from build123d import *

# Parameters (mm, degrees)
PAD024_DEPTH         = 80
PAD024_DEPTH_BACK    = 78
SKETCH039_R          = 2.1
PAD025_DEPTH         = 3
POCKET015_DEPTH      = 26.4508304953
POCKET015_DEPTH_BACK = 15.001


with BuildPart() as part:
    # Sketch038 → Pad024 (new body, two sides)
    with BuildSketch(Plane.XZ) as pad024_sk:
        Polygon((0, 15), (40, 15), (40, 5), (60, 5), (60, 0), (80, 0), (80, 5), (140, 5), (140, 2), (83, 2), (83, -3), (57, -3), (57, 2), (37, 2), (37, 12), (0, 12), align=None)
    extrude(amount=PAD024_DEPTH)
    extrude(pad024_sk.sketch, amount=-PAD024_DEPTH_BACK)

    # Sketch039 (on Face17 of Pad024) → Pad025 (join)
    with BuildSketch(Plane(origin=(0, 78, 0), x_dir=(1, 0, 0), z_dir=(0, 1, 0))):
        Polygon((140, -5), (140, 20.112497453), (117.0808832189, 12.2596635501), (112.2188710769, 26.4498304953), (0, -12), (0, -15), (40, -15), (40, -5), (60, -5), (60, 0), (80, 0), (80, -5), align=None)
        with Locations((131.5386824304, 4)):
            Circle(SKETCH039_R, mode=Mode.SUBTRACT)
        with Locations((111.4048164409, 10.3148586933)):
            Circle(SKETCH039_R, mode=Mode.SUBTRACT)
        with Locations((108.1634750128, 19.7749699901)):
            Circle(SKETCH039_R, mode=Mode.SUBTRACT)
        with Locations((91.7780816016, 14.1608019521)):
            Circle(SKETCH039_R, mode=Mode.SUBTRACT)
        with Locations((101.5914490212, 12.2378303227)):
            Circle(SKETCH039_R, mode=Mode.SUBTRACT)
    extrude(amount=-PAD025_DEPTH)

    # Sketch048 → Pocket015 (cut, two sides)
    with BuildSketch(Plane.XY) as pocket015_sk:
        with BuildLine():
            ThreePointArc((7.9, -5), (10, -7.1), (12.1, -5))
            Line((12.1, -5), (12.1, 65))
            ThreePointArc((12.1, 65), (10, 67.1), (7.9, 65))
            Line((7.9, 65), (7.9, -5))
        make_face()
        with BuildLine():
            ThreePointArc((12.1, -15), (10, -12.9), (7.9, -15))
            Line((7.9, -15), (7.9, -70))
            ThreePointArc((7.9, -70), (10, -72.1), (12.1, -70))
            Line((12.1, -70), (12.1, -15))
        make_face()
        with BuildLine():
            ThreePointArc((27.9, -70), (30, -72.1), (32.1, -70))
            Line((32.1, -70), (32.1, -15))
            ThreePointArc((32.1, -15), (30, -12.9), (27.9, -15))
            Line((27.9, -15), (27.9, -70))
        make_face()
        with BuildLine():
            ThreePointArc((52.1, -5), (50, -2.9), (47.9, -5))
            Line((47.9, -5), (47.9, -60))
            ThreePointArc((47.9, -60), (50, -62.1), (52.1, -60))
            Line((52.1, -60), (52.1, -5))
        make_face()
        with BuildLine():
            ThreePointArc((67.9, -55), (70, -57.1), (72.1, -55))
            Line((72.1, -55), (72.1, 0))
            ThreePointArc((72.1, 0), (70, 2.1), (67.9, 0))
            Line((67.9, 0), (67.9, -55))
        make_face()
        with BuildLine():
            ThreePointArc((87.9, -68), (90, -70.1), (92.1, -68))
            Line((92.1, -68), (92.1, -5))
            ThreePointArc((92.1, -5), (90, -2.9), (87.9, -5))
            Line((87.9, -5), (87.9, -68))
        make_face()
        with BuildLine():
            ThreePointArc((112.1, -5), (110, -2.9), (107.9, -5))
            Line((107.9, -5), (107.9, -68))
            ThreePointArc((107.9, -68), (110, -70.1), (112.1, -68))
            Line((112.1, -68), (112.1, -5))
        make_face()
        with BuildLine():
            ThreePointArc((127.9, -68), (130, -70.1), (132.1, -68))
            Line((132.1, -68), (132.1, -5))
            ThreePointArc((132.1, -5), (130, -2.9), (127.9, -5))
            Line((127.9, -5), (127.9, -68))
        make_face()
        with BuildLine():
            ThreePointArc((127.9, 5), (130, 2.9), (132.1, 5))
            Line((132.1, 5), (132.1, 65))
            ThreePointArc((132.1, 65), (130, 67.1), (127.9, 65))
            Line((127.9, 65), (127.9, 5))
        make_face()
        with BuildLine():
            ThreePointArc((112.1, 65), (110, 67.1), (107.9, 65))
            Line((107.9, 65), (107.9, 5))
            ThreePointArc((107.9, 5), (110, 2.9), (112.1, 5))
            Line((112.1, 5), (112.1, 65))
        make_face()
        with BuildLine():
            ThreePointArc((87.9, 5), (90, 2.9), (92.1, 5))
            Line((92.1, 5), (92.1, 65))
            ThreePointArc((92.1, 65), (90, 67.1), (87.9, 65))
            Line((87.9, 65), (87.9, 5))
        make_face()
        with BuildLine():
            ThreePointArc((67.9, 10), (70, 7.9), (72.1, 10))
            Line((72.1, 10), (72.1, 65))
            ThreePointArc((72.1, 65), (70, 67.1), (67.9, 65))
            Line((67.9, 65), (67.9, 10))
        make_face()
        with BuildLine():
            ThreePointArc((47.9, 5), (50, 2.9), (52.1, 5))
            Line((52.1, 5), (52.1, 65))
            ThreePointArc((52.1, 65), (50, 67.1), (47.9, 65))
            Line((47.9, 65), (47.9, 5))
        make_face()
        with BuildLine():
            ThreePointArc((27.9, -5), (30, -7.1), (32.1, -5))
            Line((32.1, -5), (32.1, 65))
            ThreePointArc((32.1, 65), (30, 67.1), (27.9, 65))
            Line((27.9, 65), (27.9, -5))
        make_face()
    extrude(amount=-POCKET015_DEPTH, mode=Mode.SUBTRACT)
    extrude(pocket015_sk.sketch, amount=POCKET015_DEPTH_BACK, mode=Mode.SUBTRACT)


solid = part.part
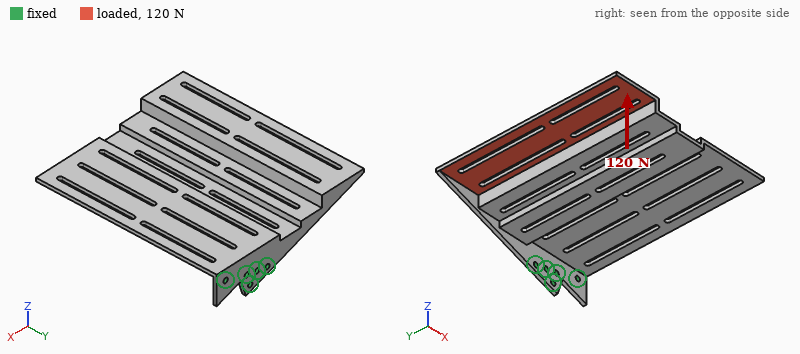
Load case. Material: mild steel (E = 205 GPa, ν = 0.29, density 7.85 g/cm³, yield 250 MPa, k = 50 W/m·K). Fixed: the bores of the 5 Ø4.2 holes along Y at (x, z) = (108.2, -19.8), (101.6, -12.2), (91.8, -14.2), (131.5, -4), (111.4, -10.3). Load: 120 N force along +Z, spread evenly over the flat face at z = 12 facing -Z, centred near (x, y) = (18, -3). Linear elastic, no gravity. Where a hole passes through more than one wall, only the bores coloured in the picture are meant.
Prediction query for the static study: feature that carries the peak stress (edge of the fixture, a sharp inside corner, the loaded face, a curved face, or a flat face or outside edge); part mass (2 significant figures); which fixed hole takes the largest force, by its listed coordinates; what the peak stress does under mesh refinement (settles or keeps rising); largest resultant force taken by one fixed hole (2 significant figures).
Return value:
edge of the fixture
550 g
(91.8, -14.2)
keeps rising
530 N
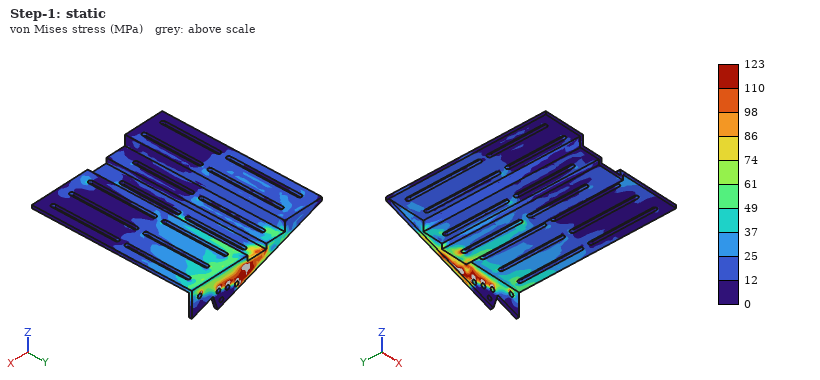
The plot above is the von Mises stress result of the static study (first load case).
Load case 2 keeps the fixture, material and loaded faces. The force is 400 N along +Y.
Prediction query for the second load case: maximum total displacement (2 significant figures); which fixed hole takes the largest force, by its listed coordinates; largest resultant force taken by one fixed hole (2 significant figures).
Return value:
1.7 mm
(131.5, -4)
860 N
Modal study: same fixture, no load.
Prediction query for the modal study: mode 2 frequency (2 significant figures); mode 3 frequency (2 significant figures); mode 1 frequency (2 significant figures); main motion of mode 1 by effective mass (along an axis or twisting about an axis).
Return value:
240 Hz
320 Hz
82 Hz
along Z
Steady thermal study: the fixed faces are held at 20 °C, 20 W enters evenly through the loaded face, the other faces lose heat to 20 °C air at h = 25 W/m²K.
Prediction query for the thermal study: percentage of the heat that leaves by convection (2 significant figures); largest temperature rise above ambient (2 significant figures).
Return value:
95 %
69 K
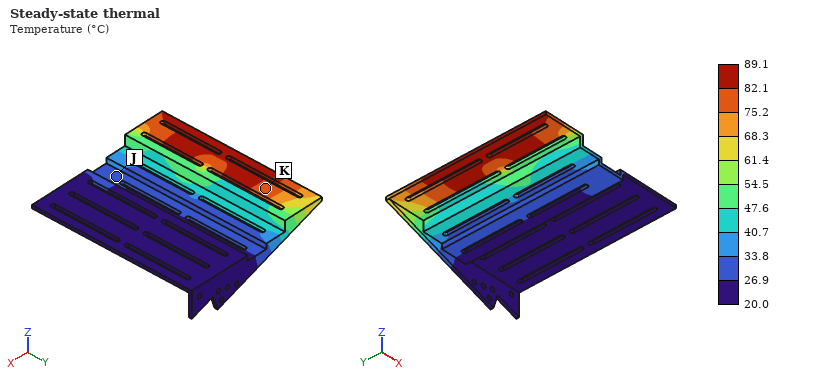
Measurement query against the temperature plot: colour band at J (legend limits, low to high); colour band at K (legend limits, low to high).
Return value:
26.9 to 33.8 °C
75.2 to 82.1 °C
